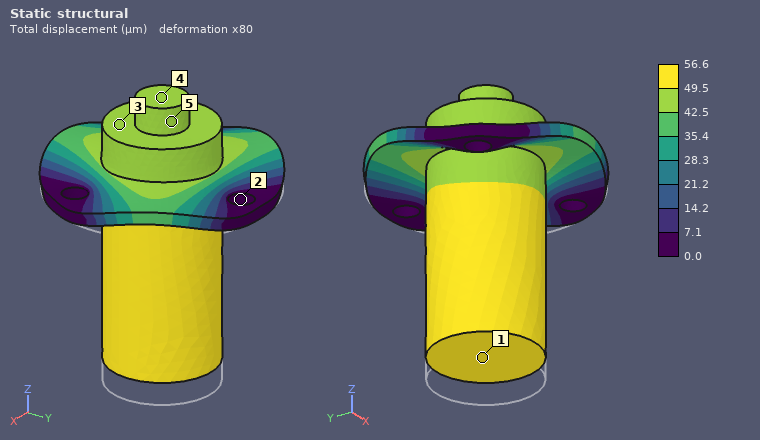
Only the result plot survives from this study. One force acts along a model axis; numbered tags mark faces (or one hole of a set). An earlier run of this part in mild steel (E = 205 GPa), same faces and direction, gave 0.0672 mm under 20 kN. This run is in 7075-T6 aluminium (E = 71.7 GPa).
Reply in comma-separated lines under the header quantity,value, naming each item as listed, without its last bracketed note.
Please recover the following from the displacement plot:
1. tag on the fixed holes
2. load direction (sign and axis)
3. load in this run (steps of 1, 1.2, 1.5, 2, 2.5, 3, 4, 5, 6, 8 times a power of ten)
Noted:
quantity,value
tag on the fixed holes,2
load direction,+Z
load in this run,6 kN
